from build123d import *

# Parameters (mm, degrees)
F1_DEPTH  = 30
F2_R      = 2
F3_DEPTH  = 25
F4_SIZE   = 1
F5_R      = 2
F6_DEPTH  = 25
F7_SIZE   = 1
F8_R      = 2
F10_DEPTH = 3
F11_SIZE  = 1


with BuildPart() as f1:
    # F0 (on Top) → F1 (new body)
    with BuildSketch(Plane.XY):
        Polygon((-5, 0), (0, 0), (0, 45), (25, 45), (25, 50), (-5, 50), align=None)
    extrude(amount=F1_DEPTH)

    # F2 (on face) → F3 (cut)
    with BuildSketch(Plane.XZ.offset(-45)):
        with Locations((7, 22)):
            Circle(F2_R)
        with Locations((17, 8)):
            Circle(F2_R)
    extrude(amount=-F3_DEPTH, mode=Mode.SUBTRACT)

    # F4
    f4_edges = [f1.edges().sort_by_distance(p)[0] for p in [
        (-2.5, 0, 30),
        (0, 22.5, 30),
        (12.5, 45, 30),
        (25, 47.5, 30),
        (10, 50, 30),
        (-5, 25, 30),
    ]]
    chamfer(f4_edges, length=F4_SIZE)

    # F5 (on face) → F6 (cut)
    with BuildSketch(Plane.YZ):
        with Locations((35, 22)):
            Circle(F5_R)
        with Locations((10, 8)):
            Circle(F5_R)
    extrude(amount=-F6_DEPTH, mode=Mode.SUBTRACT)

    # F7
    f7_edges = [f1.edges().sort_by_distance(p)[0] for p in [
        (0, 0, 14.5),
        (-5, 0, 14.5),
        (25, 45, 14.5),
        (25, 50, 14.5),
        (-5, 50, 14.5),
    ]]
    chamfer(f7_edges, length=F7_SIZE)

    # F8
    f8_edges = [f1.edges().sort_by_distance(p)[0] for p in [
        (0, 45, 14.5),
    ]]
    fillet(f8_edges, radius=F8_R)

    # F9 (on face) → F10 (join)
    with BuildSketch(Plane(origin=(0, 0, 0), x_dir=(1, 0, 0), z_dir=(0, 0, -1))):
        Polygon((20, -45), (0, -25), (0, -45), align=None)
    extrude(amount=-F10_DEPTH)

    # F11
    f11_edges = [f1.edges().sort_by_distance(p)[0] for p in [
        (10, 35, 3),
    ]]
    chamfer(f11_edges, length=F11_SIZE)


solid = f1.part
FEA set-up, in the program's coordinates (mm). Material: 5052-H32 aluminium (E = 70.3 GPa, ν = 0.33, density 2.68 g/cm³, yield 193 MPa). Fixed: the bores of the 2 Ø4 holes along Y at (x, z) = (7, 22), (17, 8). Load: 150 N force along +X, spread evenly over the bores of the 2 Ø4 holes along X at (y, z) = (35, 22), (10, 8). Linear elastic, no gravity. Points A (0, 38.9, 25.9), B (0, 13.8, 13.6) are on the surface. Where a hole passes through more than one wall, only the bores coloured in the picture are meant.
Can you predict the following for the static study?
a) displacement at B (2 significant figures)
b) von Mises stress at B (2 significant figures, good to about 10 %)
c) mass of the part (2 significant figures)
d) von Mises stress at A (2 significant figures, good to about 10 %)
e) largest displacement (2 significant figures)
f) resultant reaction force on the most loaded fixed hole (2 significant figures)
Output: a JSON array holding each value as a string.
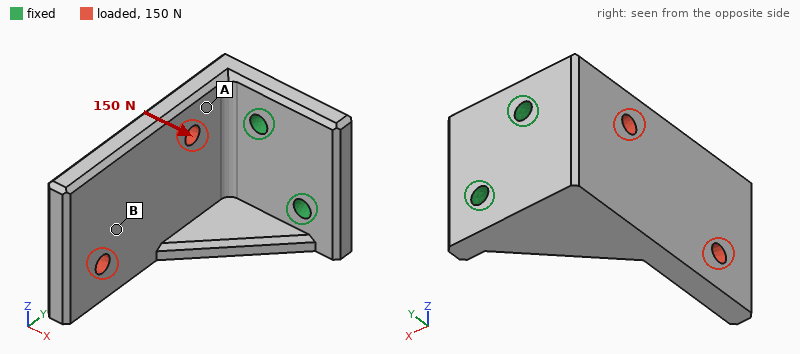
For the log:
["58 µm", "4.2 MPa", "31 g", "12 MPa", "94 µm", "110 N"]
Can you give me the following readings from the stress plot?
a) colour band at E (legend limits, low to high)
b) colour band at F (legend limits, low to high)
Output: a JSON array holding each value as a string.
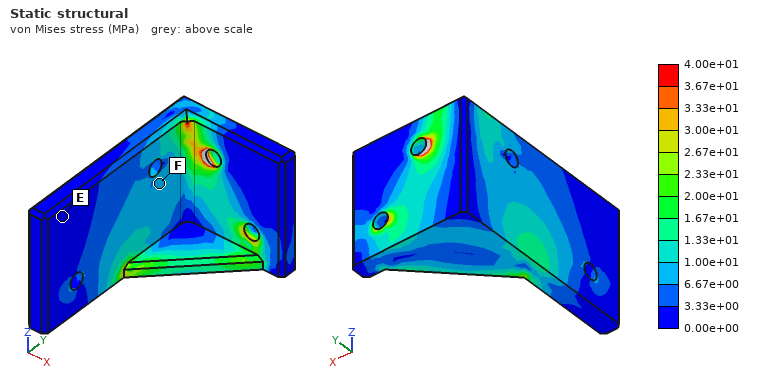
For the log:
["0.00e+00 to 3.33e+00 MPa", "6.67e+00 to 1.00e+01 MPa"]
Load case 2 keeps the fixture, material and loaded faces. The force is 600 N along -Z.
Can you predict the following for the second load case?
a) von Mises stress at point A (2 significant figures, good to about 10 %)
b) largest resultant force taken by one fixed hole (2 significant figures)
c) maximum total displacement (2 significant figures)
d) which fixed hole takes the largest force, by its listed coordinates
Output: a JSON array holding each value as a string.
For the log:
["36 MPa", "840 N", "0.19 mm", "(7, 22)"]
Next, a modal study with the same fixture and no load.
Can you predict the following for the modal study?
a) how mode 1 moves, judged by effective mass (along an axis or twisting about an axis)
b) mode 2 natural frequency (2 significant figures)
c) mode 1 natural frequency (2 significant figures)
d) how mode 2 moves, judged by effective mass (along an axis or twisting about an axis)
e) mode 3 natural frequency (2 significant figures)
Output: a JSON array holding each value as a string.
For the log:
["along X", "3200 Hz", "1800 Hz", "along Z", "7400 Hz"]
